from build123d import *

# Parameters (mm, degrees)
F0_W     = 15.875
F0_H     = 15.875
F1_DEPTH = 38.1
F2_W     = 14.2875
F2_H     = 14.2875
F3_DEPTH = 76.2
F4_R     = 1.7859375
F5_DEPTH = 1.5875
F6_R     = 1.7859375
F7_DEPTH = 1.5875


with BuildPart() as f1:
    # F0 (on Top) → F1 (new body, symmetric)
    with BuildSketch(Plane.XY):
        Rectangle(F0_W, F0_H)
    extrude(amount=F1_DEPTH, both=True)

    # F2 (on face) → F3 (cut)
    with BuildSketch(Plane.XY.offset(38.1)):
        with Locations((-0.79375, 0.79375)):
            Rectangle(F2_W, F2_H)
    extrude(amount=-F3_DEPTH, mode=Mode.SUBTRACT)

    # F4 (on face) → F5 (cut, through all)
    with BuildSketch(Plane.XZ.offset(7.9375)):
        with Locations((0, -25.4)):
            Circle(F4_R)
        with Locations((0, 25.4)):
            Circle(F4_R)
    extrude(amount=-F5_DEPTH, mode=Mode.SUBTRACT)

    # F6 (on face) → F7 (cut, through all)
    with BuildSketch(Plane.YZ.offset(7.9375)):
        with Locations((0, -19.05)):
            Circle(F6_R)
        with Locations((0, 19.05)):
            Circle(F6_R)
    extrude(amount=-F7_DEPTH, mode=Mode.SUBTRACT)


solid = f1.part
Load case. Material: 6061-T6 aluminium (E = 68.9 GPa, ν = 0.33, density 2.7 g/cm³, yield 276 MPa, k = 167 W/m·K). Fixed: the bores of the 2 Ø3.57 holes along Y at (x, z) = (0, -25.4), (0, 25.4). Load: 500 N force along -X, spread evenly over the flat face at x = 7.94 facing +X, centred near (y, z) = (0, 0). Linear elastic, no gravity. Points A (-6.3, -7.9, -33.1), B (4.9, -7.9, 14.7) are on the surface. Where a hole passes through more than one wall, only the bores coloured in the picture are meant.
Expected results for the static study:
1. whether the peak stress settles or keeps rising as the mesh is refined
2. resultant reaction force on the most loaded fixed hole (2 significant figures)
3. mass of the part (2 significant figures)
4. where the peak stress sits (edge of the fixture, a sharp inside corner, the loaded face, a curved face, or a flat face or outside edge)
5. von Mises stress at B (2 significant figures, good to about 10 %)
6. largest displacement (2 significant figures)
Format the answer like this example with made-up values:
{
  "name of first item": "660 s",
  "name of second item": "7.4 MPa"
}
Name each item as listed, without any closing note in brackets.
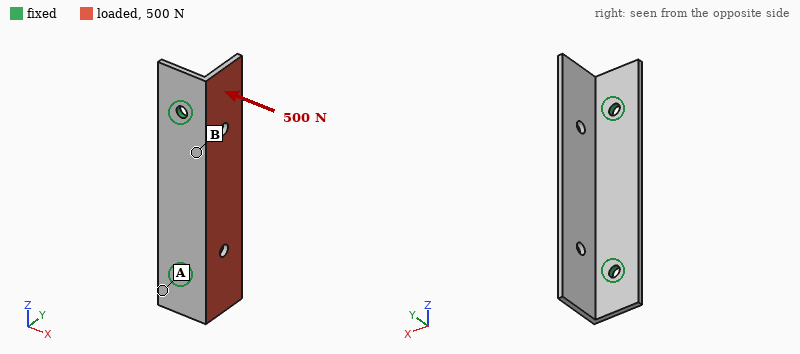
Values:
{
  "whether the peak stress settles or keeps rising as the mesh is refined": "keeps rising",
  "resultant reaction force on the most loaded fixed hole": "250 N",
  "mass of the part": "9.7 g",
  "where the peak stress sits": "edge of the fixture",
  "von Mises stress at B": "91 MPa",
  "largest displacement": "0.45 mm"
}
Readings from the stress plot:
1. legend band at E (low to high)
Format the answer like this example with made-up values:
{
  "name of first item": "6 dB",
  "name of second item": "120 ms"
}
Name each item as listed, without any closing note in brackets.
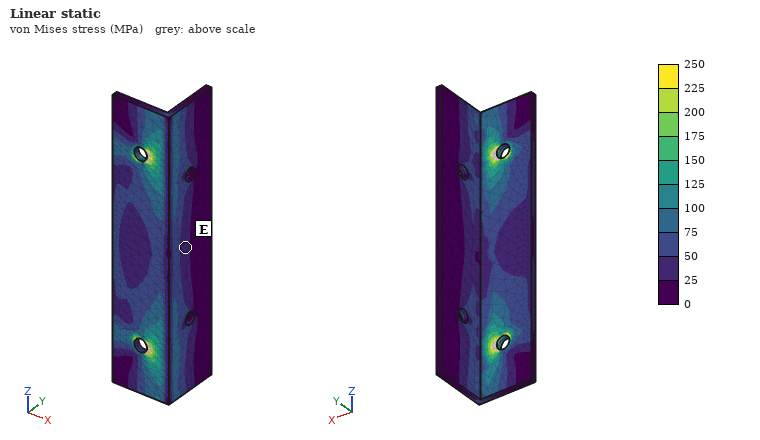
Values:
{
  "legend band at E": "25 to 50 MPa"
}
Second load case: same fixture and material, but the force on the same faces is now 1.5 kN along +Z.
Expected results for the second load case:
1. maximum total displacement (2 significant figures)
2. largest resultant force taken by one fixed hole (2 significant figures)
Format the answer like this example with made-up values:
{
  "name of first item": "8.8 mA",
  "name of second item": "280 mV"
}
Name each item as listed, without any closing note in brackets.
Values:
{
  "maximum total displacement": "95 µm",
  "largest resultant force taken by one fixed hole": "800 N"
}
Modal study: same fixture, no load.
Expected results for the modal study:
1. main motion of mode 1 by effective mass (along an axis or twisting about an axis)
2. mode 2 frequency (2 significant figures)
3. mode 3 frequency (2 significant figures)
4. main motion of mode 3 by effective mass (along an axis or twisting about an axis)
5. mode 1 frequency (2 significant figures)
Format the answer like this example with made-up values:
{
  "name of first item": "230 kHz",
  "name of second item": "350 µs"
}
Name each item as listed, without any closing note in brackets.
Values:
{
  "main motion of mode 1 by effective mass": "along X",
  "mode 2 frequency": "3900 Hz",
  "mode 3 frequency": "5000 Hz",
  "main motion of mode 3 by effective mass": "along Y",
  "mode 1 frequency": "2800 Hz"
}
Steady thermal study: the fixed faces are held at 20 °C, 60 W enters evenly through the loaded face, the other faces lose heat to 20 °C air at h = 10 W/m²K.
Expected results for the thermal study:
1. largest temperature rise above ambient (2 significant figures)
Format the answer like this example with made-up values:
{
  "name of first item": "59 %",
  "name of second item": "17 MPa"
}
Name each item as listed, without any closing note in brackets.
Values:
{
  "largest temperature rise above ambient": "75 K"
}
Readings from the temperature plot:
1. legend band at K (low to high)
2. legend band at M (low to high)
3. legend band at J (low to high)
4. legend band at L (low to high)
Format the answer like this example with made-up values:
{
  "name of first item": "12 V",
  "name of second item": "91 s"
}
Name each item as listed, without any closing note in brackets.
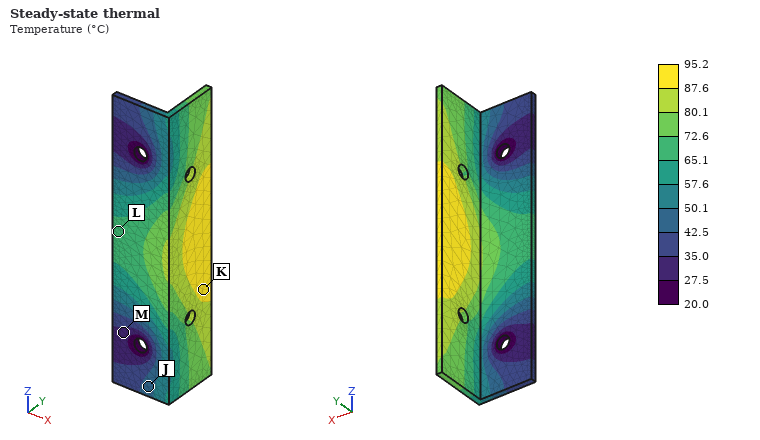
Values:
{
  "legend band at K": "87.6 to 95.2 °C",
  "legend band at M": "27.5 to 35.0 °C",
  "legend band at J": "42.5 to 50.1 °C",
  "legend band at L": "65.1 to 72.6 °C"
}
